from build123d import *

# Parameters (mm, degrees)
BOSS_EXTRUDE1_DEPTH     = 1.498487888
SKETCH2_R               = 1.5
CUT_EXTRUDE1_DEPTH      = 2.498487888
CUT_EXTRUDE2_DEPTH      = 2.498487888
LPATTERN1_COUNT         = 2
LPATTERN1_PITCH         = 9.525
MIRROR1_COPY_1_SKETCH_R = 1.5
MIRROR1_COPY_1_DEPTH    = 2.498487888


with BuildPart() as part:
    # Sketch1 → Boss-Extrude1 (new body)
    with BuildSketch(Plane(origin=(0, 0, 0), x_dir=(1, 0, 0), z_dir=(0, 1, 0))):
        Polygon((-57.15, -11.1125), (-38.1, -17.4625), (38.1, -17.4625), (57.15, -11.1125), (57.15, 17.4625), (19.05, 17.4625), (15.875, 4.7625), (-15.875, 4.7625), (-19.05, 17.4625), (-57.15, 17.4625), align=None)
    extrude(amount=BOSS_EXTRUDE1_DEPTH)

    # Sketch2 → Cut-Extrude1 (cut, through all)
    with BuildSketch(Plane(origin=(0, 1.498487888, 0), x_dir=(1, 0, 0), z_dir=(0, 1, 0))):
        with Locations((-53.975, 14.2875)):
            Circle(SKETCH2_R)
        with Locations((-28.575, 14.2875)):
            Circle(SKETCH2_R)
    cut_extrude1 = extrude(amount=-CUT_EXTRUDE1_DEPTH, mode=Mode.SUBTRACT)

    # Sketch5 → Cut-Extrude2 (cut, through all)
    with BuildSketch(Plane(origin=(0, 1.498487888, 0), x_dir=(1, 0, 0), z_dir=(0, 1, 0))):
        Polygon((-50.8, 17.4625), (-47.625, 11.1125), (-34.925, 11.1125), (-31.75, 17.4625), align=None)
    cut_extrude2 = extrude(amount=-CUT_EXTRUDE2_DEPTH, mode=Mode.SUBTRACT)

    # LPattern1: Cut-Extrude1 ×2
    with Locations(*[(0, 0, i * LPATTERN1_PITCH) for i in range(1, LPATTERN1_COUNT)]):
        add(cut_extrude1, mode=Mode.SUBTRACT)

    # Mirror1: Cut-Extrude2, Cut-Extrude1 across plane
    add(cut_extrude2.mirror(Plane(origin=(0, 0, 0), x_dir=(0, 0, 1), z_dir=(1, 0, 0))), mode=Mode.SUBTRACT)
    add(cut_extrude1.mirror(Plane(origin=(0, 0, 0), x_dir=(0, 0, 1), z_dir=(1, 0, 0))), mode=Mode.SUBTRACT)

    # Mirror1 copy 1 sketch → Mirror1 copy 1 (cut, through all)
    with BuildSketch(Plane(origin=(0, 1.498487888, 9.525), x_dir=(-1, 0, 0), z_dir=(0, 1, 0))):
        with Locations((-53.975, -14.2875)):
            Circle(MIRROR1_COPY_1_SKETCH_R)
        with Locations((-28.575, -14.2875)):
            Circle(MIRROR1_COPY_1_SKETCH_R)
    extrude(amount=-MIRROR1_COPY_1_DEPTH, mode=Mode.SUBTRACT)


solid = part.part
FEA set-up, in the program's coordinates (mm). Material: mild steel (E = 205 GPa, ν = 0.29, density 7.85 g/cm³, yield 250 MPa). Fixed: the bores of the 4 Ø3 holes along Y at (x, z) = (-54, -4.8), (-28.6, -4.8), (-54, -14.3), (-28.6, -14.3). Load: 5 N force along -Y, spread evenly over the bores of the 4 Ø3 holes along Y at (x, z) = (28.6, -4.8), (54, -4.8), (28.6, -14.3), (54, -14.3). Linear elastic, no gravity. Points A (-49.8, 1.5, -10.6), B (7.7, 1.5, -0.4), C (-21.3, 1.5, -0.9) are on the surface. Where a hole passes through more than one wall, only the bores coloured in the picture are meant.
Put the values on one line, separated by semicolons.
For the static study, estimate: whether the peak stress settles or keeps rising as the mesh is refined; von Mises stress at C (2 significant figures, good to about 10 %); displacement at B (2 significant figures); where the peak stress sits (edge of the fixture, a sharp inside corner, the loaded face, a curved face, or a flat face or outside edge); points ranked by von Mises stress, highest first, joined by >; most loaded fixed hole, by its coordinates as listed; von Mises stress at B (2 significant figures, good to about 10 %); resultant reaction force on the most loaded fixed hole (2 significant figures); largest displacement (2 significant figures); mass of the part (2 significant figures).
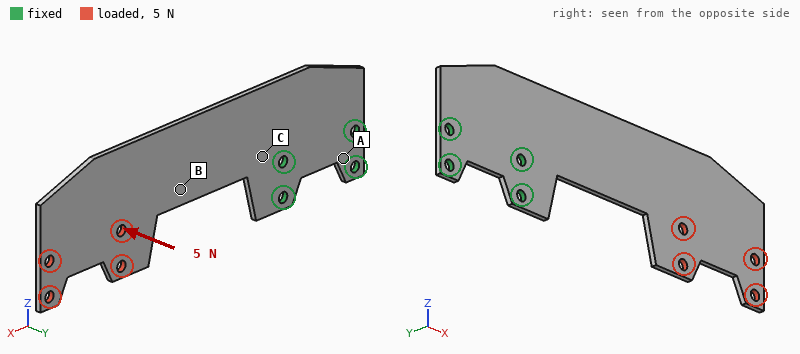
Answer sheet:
keeps rising; 31 MPa; 0.14 mm; edge of the fixture; C > B > A; (-28.6, -4.8); 23 MPa; 10 N; 0.61 mm; 37 g
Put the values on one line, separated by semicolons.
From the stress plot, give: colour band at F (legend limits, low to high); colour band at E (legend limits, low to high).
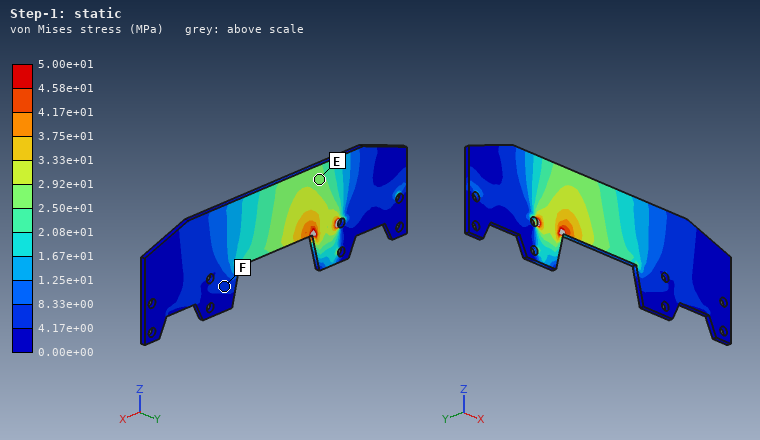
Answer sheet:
4.17e+00 to 8.33e+00 MPa; 2.50e+01 to 2.92e+01 MPa
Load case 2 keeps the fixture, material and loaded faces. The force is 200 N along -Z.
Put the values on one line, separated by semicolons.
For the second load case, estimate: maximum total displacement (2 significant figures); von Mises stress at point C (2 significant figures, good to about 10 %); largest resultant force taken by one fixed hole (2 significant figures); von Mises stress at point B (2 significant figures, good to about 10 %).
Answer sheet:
0.12 mm; 29 MPa; 440 N; 34 MPa
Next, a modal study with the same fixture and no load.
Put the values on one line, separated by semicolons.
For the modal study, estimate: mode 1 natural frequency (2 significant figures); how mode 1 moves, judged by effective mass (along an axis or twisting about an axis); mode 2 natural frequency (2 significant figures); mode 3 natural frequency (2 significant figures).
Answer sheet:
150 Hz; along Y; 750 Hz; 1000 Hz
